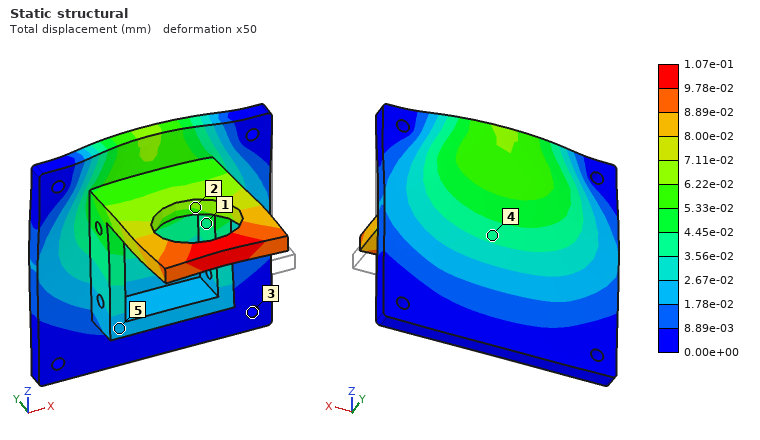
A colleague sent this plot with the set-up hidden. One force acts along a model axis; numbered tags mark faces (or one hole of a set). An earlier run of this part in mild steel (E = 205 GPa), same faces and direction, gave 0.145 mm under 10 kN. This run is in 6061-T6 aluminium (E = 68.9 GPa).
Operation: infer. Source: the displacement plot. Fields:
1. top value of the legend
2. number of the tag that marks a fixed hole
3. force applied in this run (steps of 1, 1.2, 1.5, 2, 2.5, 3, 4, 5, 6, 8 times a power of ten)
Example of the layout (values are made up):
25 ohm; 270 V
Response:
1.07e-01 mm; 3; 2.5 kN
